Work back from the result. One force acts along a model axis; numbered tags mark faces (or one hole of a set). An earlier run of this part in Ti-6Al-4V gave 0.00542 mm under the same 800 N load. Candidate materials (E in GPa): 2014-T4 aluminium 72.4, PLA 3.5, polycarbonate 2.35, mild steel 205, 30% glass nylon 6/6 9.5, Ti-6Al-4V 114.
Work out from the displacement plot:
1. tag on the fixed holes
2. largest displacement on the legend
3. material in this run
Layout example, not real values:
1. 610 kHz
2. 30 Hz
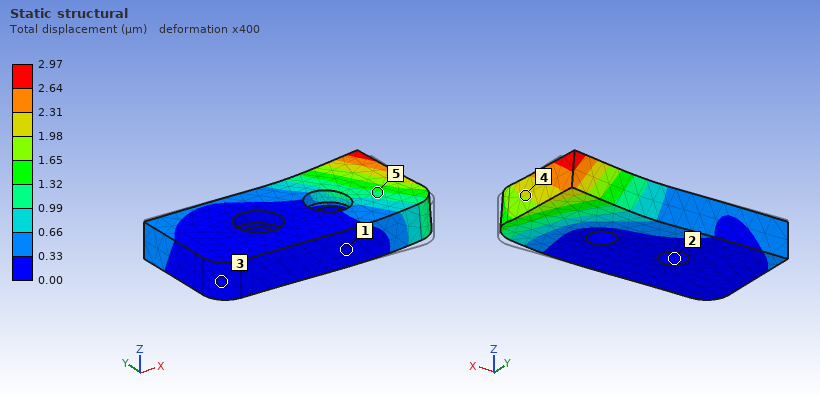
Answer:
1. 2
2. 2.97 µm
3. mild steel
